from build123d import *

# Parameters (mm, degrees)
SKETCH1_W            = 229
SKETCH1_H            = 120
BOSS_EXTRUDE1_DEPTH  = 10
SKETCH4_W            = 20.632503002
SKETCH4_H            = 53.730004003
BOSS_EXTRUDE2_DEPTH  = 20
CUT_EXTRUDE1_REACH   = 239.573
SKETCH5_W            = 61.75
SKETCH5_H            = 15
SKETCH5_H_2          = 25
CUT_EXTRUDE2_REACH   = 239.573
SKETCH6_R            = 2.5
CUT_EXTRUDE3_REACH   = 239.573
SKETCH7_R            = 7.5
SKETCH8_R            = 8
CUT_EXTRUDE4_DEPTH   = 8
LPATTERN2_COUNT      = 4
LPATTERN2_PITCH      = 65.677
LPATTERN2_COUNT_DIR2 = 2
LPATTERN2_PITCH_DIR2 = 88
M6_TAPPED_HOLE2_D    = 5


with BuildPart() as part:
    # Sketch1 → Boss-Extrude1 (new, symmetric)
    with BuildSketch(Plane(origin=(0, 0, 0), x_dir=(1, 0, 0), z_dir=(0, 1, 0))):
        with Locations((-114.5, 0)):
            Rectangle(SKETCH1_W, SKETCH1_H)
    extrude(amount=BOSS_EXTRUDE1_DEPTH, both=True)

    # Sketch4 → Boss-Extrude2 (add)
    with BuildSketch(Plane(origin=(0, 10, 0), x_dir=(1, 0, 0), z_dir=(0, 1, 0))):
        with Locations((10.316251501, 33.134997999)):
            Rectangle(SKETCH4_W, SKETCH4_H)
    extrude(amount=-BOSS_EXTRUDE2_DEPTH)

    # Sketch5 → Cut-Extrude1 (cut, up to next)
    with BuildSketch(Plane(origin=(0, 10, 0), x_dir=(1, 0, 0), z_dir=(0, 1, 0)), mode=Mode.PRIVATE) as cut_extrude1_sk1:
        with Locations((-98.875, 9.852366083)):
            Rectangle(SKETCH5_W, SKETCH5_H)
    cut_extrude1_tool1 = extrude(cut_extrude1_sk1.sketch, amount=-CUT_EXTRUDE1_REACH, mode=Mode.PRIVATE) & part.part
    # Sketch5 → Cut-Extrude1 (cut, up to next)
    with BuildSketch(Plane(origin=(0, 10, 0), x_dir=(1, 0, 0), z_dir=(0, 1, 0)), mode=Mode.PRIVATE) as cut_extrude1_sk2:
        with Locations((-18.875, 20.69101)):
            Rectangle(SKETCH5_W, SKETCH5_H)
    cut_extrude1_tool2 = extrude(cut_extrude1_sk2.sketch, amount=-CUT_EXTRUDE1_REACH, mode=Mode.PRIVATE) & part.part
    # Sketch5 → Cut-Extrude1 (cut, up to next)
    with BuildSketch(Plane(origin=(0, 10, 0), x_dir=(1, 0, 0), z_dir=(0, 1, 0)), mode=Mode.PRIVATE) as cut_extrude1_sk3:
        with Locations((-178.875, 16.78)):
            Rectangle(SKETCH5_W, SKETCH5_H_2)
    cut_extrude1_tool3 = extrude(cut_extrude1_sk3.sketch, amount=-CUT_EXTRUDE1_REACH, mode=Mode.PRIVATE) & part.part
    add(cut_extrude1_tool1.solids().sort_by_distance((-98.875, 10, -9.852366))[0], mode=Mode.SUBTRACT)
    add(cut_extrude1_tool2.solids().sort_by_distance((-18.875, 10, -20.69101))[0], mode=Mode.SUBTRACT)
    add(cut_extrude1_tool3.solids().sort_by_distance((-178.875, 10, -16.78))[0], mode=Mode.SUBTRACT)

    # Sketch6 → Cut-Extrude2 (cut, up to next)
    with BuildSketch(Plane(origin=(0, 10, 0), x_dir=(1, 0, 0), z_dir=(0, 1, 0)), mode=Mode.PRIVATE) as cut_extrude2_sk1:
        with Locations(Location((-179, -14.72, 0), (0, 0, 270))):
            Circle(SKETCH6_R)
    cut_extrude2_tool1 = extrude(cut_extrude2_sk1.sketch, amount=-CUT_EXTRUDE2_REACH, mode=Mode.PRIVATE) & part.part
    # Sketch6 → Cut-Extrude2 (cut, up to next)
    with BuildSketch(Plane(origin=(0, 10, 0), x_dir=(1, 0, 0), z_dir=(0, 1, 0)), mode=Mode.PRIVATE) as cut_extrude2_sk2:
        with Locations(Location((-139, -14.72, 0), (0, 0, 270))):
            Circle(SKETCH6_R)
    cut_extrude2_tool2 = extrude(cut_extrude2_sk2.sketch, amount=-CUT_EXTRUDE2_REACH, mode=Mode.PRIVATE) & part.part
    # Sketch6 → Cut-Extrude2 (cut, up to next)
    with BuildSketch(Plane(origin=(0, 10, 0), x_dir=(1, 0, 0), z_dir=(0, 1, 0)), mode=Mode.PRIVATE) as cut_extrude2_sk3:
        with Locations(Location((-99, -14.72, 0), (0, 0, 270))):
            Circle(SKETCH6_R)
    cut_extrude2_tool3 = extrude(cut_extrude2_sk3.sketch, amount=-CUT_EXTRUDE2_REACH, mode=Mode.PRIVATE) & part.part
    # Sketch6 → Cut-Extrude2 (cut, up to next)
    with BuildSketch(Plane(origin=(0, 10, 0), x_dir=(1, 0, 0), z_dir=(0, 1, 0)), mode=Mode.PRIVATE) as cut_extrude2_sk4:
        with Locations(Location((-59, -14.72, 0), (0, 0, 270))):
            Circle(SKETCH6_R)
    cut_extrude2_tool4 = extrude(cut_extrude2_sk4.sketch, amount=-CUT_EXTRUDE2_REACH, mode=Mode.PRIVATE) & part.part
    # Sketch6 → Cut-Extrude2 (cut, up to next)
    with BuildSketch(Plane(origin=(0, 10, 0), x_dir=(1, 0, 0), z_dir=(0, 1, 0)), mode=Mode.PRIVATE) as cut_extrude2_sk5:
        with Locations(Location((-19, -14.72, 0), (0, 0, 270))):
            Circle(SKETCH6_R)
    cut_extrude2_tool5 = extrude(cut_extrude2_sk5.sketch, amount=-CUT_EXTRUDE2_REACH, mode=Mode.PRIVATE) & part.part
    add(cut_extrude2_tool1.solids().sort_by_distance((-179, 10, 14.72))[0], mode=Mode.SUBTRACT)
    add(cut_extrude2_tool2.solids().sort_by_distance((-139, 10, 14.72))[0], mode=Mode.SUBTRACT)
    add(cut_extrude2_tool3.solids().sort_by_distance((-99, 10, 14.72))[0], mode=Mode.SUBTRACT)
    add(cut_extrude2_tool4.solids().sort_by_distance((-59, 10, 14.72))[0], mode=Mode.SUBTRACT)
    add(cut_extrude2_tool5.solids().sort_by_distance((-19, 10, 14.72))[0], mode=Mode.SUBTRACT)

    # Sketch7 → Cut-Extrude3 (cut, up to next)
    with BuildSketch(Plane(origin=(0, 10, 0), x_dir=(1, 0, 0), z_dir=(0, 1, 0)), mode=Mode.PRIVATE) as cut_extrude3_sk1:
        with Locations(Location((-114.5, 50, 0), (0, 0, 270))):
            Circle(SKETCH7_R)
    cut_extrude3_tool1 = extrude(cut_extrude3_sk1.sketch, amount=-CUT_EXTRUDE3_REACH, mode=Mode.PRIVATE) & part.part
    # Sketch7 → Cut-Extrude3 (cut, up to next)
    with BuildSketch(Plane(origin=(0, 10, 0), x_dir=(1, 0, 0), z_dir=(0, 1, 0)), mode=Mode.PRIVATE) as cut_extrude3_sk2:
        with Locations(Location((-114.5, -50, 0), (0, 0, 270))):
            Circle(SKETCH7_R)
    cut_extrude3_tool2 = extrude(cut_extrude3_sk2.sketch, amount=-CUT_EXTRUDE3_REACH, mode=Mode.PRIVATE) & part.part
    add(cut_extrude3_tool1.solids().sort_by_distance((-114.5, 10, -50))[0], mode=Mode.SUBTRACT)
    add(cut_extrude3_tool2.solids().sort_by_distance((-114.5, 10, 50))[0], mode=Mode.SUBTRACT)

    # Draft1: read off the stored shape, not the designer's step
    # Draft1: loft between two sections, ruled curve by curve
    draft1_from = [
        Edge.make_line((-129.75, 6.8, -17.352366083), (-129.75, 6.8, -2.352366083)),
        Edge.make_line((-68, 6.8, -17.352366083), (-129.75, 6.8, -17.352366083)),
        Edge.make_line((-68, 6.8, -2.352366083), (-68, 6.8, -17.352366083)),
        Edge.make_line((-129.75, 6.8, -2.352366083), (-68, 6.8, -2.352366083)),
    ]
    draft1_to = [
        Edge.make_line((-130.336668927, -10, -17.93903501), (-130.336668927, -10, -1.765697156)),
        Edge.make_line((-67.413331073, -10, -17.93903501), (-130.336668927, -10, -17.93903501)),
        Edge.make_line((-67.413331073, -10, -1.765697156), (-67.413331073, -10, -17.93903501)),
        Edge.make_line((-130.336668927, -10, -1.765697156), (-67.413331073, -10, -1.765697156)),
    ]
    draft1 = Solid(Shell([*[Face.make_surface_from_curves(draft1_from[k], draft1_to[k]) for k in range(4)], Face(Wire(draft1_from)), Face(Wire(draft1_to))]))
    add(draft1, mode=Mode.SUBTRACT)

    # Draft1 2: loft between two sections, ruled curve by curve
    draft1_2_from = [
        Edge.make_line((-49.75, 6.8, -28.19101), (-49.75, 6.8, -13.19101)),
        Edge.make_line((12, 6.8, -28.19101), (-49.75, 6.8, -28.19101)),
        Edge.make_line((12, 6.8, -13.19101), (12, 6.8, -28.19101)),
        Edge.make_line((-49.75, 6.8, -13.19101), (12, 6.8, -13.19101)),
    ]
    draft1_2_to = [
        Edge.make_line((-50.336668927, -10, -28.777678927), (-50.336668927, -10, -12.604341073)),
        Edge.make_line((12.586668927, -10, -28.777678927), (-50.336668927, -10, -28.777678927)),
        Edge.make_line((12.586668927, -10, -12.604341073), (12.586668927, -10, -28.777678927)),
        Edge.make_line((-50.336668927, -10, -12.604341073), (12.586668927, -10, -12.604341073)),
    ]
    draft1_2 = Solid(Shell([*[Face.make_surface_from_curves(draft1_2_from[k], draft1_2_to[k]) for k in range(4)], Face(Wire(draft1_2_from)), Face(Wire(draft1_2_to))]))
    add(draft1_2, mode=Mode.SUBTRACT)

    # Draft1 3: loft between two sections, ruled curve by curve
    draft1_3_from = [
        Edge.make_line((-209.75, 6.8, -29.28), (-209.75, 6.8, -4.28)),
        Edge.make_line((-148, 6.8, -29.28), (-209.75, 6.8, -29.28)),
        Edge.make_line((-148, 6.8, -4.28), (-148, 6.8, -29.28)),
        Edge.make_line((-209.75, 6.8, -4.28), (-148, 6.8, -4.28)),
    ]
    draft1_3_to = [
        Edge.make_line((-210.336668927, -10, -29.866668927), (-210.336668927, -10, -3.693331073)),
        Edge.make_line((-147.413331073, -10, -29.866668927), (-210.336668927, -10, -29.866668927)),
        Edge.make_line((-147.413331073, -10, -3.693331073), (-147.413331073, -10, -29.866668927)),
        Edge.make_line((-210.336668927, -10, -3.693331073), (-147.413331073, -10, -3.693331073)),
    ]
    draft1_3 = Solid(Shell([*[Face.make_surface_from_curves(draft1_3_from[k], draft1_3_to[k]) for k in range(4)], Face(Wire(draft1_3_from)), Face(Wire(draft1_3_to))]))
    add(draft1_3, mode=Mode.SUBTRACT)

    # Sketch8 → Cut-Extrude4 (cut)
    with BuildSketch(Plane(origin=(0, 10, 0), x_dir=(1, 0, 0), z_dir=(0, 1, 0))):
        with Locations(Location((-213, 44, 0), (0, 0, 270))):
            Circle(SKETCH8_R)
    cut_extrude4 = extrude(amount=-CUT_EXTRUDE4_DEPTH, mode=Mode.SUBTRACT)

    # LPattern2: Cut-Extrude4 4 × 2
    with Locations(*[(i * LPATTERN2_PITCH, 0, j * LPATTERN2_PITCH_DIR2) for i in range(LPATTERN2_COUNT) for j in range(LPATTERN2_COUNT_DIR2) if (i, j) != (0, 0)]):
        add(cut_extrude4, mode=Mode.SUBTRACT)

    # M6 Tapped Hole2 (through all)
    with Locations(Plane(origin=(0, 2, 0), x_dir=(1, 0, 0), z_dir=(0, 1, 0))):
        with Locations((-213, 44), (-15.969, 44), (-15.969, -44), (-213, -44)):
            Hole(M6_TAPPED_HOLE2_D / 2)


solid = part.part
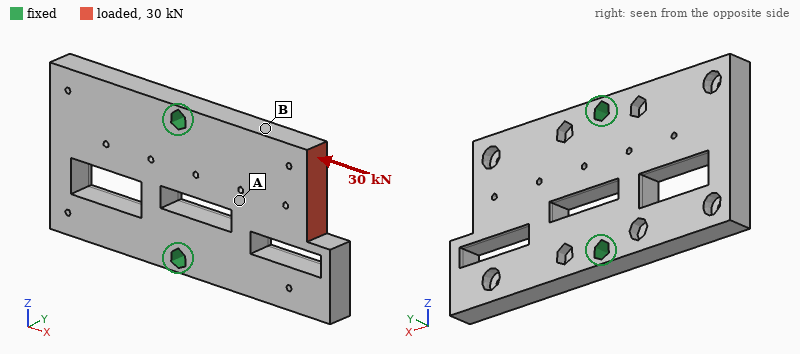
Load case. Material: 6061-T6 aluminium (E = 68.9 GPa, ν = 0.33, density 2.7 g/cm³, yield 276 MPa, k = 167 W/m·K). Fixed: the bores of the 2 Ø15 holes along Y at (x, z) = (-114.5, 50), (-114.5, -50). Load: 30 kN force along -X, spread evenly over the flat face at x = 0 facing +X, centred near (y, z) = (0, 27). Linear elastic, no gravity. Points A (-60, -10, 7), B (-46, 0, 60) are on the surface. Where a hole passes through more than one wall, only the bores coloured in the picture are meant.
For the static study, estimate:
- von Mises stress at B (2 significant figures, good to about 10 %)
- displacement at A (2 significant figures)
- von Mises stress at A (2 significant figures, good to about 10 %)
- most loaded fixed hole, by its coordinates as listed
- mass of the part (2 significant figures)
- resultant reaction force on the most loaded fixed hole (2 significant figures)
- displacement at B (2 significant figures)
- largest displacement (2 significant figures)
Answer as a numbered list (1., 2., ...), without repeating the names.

1. 29 MPa
2. 20 µm
3. 13 MPa
4. (-114.5, 50)
5. 1.3 kg
6. 24 kN
7. 33 µm
8. 62 µm
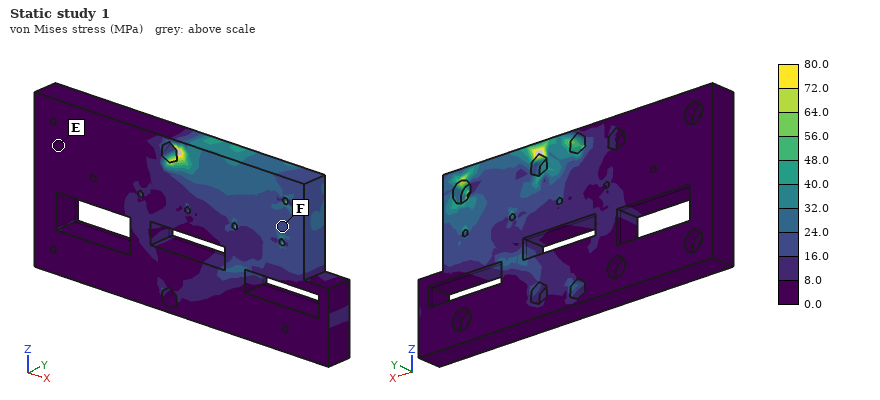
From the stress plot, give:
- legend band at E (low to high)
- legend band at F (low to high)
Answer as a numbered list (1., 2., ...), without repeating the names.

1. 0.0 to 8.0 MPa
2. 16.0 to 24.0 MPa
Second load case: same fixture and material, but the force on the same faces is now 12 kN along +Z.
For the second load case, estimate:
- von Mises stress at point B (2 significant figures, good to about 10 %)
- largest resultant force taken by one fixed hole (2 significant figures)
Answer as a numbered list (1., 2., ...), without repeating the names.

1. 23 MPa
2. 14 kN
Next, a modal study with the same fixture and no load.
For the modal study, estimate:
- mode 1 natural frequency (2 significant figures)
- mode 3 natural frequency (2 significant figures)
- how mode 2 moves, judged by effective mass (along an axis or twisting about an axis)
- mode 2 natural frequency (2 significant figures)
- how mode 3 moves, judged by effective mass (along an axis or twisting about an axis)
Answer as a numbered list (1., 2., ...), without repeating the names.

1. 960 Hz
2. 2200 Hz
3. along Y
4. 1200 Hz
5. twisting about X
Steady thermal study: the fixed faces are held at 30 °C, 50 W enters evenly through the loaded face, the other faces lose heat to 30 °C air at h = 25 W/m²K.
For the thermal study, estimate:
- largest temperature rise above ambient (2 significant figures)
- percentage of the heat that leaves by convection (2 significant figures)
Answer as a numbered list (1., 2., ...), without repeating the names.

1. 22 K
2. 18 %
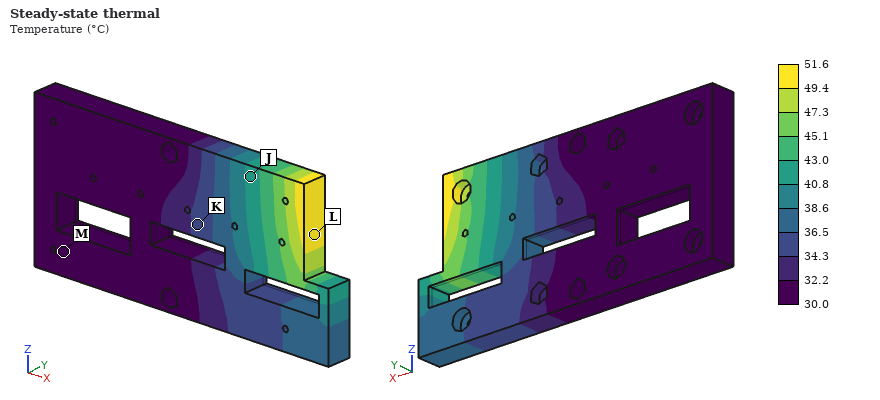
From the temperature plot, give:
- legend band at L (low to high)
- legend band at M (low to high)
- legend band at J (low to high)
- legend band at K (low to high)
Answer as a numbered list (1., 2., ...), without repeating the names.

1. 49.4 to 51.6 °C
2. 30.0 to 32.2 °C
3. 40.8 to 43.0 °C
4. 34.3 to 36.5 °C
